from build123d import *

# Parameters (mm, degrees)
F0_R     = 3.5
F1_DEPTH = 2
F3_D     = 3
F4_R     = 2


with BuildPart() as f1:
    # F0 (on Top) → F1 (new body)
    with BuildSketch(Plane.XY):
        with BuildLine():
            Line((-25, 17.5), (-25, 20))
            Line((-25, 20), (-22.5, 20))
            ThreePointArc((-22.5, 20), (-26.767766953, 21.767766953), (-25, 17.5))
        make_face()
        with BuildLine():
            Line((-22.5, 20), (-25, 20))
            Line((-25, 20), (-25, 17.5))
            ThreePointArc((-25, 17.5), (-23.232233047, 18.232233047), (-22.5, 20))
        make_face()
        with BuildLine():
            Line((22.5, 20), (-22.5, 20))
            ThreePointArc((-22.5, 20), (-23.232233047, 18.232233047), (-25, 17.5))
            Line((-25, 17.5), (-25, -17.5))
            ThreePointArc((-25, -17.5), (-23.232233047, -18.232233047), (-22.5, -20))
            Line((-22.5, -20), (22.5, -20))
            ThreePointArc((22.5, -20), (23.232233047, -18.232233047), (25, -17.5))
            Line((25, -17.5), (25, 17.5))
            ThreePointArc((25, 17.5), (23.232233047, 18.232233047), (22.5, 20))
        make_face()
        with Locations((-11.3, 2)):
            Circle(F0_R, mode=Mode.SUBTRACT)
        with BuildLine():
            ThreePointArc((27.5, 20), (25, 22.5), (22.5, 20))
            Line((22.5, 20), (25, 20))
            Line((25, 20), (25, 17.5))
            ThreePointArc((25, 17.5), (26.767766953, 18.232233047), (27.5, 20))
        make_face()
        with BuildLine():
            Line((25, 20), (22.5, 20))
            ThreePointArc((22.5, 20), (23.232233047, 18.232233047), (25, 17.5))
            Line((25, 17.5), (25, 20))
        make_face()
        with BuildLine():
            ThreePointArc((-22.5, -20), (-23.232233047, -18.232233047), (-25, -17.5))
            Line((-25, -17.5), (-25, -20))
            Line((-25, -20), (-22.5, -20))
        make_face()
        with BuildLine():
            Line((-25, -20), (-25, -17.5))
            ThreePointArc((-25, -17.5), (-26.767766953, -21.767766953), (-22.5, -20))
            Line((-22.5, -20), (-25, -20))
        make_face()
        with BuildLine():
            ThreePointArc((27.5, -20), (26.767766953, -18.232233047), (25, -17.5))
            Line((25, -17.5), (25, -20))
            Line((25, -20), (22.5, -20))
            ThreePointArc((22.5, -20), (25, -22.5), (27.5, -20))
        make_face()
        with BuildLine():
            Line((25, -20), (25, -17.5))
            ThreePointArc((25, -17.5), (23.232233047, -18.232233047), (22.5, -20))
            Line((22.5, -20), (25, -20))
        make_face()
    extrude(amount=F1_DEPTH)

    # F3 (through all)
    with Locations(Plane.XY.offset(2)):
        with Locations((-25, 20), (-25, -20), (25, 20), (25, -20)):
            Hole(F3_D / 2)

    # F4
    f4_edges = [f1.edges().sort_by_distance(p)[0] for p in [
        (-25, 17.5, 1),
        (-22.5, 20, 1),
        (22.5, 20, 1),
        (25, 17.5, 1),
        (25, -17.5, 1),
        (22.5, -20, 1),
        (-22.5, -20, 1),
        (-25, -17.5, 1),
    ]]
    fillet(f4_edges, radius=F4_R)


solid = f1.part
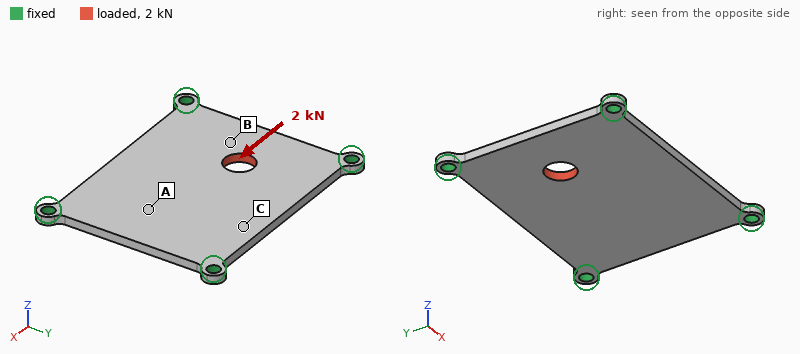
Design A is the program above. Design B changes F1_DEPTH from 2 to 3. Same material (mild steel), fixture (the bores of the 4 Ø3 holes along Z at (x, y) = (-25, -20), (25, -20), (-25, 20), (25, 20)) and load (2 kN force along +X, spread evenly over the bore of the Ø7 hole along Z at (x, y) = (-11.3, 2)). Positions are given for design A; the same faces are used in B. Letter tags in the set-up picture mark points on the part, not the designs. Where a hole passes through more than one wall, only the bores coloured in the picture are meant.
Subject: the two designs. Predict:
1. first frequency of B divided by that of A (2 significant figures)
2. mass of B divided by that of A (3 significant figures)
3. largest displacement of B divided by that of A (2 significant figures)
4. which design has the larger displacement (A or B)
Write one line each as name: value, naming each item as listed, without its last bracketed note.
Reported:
first frequency of B divided by that of A: 1.5
mass of B divided by that of A: 1.50
largest displacement of B divided by that of A: 0.67
which design has the larger displacement: A
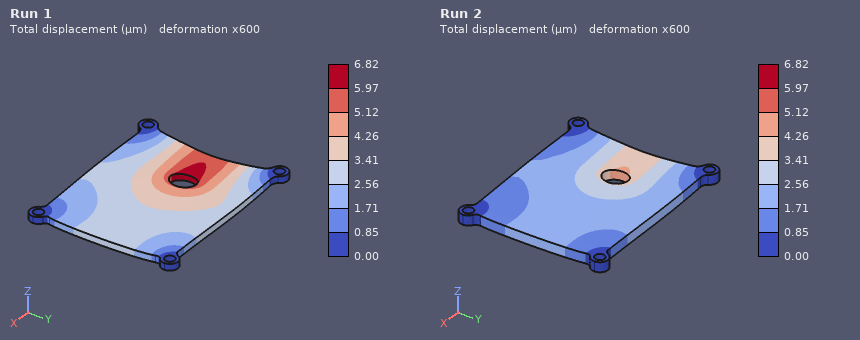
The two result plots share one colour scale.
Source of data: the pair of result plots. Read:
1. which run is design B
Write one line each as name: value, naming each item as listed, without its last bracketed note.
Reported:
which run is design B: Run 2
